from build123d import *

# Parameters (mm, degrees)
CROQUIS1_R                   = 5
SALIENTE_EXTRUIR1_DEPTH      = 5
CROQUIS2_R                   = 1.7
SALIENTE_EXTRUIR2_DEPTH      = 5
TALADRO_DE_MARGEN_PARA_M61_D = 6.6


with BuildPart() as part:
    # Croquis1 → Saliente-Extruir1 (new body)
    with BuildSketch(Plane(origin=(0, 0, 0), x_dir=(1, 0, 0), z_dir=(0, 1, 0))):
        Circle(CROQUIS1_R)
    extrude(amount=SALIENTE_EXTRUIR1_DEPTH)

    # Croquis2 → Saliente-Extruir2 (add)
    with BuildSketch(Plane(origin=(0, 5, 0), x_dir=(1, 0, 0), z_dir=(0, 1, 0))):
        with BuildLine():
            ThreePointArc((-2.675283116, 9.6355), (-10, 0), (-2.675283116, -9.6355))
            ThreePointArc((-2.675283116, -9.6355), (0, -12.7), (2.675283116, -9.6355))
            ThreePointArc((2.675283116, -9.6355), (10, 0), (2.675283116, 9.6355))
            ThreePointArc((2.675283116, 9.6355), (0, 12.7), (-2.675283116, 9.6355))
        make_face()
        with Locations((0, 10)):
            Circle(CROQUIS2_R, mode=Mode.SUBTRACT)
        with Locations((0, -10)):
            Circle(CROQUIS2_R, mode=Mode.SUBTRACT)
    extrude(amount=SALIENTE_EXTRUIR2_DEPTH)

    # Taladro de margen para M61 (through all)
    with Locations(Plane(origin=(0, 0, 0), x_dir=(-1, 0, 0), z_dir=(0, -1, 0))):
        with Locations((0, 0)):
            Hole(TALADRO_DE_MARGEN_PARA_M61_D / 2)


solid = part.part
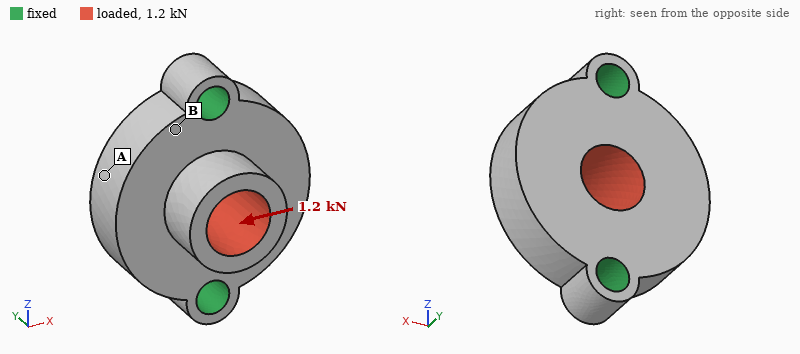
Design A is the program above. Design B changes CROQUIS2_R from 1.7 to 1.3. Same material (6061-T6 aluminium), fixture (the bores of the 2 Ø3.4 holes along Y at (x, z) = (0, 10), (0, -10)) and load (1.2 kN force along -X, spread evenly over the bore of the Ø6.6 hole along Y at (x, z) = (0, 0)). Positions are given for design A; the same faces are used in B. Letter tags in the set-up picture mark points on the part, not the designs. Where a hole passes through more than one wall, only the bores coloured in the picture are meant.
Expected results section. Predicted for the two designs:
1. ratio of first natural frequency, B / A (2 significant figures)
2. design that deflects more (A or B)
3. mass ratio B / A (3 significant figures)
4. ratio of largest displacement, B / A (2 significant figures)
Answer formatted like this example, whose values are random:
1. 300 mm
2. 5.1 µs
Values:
1. 0.91
2. B
3. 1.02
4. 1.1
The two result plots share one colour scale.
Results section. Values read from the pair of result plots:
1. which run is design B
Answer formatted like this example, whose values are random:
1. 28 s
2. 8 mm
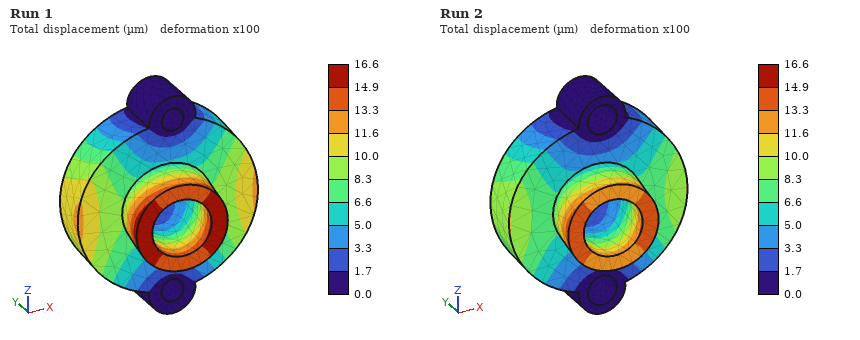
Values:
1. Run 1
